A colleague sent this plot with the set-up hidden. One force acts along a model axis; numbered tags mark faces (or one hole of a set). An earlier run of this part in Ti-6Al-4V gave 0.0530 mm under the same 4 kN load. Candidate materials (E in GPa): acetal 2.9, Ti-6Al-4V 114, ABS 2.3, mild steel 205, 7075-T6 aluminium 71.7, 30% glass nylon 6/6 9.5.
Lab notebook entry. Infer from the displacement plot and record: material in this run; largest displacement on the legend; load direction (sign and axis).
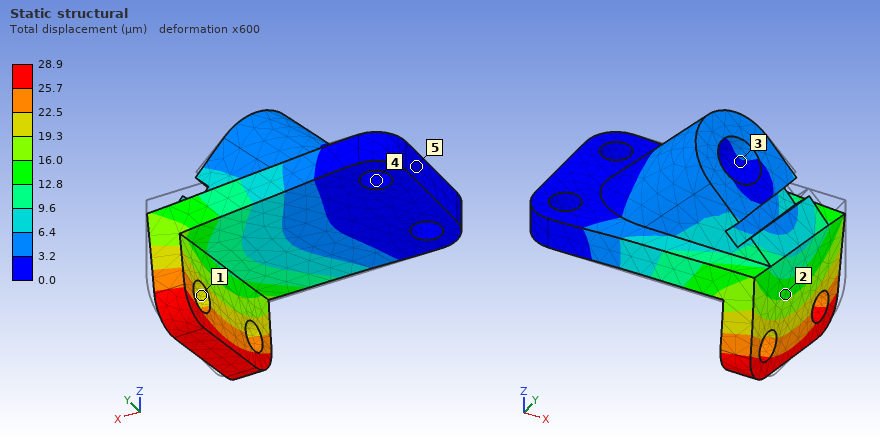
mild steel
28.9 µm
-Y
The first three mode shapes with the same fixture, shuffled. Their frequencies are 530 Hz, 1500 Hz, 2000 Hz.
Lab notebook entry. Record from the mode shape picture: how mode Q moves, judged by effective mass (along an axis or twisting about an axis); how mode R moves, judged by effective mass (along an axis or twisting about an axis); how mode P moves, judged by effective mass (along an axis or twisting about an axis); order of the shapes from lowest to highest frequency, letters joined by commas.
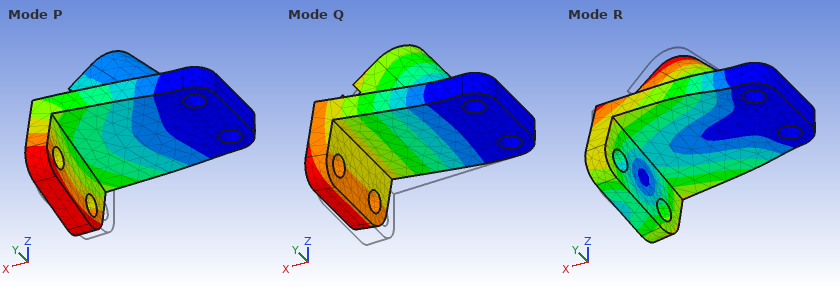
along Z
along Y
along Y
Q, P, R
